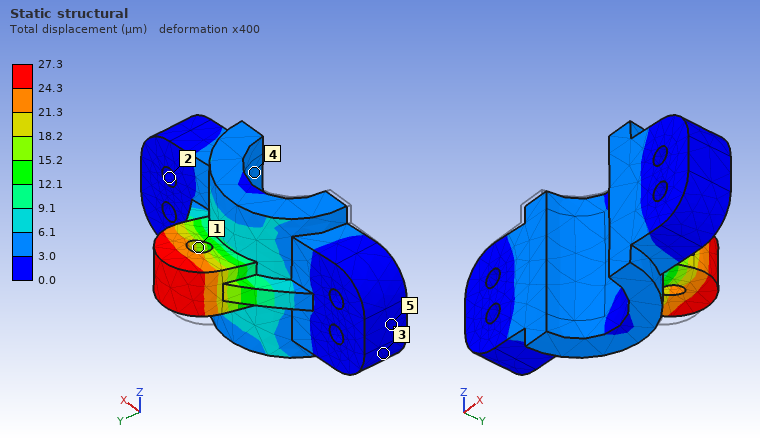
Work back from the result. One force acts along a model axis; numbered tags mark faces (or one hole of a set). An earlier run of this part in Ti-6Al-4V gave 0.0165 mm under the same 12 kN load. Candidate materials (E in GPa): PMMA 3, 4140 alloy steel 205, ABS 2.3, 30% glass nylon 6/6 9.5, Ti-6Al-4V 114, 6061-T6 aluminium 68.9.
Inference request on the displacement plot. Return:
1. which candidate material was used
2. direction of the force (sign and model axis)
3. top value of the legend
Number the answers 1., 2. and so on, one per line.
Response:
1. 6061-T6 aluminium
2. +X
3. 27.3 µm
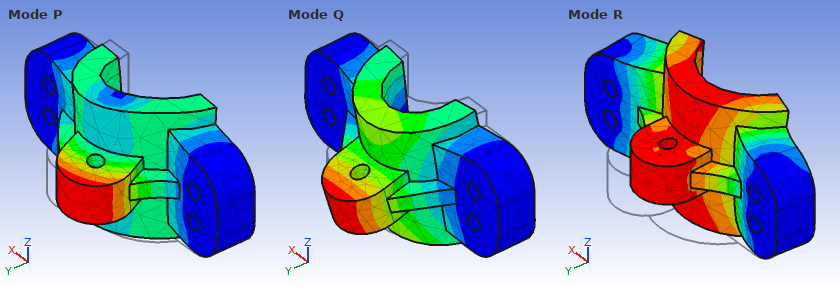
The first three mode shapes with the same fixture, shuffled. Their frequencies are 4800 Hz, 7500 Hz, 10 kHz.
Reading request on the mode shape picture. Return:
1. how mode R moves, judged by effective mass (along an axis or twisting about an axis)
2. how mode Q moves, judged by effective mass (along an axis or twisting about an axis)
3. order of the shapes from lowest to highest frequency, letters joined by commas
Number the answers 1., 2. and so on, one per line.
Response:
1. along Y
2. along Z
3. Q, R, P
